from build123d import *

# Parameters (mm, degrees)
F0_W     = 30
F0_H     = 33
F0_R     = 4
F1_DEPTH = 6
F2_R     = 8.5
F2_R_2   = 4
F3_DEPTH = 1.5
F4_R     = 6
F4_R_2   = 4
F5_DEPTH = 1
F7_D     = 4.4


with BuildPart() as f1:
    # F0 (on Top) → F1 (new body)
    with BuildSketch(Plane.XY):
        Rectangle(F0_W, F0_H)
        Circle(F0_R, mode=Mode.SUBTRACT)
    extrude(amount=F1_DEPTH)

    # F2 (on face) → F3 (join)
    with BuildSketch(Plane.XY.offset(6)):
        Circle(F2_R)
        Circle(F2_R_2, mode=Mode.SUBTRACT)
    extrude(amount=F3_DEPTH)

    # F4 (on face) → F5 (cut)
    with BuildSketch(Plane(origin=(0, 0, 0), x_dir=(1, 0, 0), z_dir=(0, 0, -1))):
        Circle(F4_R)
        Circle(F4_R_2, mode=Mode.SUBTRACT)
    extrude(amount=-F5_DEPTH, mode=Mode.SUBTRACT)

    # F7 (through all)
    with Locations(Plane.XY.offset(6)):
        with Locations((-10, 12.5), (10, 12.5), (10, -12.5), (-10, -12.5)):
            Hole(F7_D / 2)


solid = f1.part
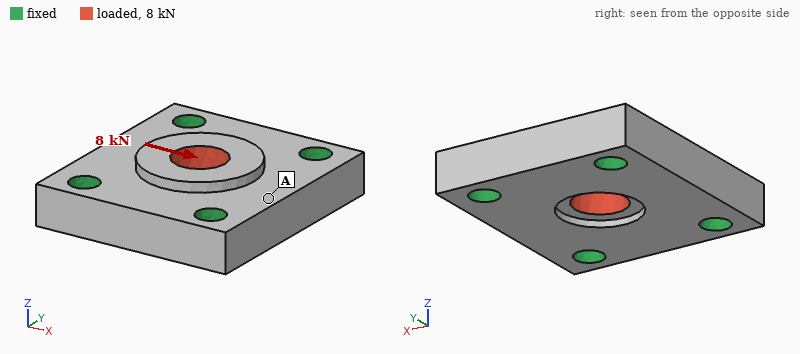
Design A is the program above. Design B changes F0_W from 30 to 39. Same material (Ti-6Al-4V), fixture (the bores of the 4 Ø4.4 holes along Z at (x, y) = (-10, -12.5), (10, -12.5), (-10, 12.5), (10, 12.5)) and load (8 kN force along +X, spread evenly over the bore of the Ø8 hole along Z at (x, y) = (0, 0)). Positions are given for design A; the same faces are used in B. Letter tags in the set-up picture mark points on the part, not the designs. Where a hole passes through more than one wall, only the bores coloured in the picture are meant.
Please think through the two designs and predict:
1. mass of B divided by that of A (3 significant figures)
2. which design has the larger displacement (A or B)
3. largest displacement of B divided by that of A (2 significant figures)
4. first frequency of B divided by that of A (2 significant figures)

1.33
A
0.90
0.88
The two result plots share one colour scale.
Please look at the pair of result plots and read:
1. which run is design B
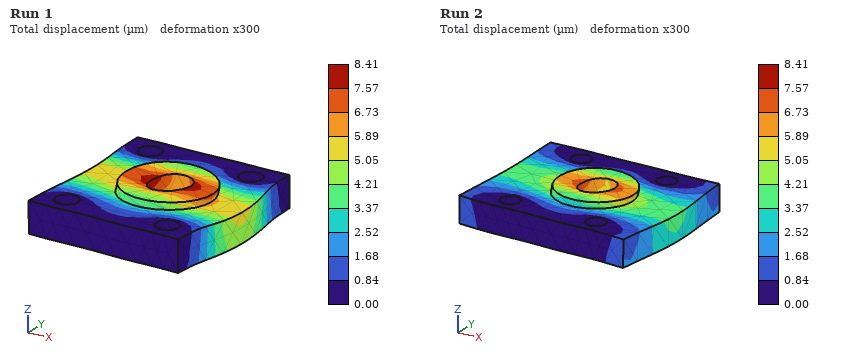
Run 2
